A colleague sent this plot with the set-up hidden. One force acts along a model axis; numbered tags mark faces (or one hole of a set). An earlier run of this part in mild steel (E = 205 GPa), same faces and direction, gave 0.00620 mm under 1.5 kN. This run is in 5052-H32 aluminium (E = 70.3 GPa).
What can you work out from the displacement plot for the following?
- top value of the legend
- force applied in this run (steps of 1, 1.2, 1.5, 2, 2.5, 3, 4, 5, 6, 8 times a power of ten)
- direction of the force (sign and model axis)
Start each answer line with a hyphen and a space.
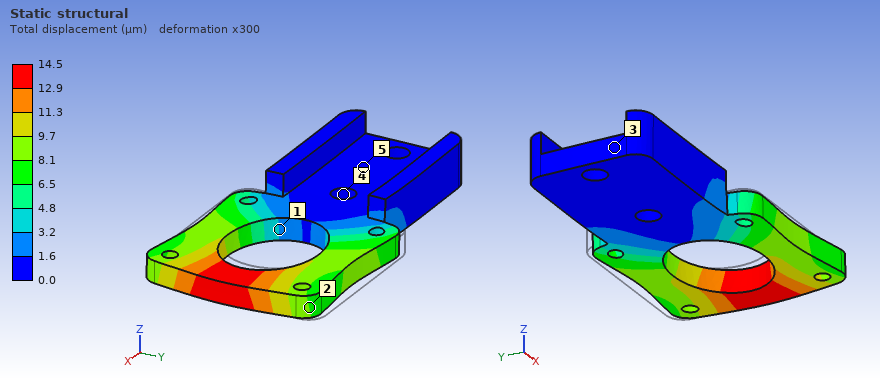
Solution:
- 14.5 µm
- 1.2 kN
- +X
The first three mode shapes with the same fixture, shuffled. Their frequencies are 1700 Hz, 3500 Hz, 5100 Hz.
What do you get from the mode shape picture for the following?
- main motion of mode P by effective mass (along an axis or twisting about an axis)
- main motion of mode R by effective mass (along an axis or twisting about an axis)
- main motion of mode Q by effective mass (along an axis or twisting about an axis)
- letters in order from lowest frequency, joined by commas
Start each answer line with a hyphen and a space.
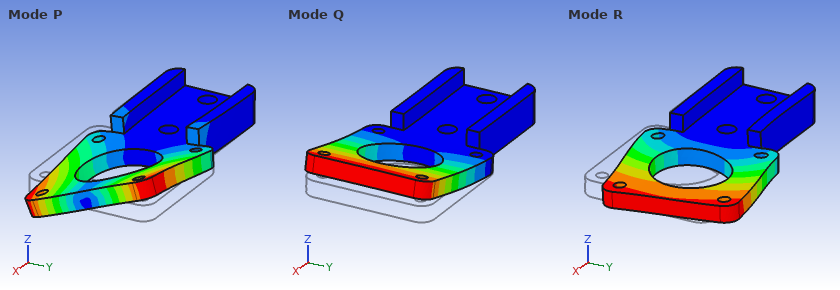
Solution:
- twisting about X
- along Y
- along Z
- Q, P, R
